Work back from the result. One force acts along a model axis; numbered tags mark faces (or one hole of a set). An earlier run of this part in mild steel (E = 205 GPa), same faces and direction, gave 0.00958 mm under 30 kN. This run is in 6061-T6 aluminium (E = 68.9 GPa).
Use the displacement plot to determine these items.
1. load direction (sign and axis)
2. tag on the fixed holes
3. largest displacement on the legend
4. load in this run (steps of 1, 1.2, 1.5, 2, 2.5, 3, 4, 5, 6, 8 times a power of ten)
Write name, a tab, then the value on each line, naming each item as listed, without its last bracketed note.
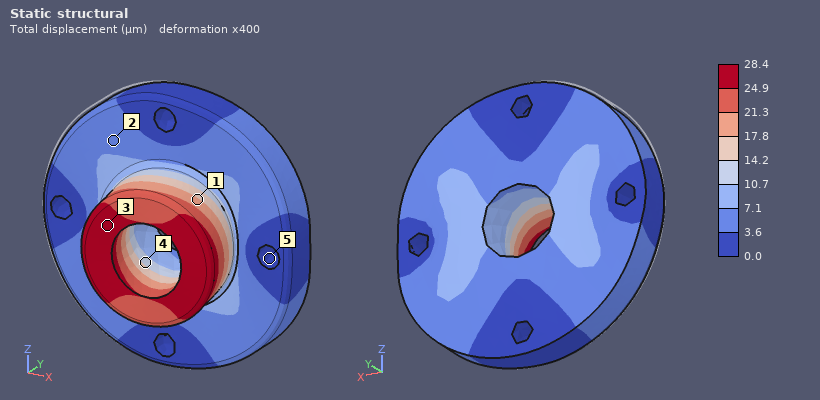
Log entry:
load direction	+X
tag on the fixed holes	5
largest displacement on the legend	28.4 µm
load in this run	30 kN
